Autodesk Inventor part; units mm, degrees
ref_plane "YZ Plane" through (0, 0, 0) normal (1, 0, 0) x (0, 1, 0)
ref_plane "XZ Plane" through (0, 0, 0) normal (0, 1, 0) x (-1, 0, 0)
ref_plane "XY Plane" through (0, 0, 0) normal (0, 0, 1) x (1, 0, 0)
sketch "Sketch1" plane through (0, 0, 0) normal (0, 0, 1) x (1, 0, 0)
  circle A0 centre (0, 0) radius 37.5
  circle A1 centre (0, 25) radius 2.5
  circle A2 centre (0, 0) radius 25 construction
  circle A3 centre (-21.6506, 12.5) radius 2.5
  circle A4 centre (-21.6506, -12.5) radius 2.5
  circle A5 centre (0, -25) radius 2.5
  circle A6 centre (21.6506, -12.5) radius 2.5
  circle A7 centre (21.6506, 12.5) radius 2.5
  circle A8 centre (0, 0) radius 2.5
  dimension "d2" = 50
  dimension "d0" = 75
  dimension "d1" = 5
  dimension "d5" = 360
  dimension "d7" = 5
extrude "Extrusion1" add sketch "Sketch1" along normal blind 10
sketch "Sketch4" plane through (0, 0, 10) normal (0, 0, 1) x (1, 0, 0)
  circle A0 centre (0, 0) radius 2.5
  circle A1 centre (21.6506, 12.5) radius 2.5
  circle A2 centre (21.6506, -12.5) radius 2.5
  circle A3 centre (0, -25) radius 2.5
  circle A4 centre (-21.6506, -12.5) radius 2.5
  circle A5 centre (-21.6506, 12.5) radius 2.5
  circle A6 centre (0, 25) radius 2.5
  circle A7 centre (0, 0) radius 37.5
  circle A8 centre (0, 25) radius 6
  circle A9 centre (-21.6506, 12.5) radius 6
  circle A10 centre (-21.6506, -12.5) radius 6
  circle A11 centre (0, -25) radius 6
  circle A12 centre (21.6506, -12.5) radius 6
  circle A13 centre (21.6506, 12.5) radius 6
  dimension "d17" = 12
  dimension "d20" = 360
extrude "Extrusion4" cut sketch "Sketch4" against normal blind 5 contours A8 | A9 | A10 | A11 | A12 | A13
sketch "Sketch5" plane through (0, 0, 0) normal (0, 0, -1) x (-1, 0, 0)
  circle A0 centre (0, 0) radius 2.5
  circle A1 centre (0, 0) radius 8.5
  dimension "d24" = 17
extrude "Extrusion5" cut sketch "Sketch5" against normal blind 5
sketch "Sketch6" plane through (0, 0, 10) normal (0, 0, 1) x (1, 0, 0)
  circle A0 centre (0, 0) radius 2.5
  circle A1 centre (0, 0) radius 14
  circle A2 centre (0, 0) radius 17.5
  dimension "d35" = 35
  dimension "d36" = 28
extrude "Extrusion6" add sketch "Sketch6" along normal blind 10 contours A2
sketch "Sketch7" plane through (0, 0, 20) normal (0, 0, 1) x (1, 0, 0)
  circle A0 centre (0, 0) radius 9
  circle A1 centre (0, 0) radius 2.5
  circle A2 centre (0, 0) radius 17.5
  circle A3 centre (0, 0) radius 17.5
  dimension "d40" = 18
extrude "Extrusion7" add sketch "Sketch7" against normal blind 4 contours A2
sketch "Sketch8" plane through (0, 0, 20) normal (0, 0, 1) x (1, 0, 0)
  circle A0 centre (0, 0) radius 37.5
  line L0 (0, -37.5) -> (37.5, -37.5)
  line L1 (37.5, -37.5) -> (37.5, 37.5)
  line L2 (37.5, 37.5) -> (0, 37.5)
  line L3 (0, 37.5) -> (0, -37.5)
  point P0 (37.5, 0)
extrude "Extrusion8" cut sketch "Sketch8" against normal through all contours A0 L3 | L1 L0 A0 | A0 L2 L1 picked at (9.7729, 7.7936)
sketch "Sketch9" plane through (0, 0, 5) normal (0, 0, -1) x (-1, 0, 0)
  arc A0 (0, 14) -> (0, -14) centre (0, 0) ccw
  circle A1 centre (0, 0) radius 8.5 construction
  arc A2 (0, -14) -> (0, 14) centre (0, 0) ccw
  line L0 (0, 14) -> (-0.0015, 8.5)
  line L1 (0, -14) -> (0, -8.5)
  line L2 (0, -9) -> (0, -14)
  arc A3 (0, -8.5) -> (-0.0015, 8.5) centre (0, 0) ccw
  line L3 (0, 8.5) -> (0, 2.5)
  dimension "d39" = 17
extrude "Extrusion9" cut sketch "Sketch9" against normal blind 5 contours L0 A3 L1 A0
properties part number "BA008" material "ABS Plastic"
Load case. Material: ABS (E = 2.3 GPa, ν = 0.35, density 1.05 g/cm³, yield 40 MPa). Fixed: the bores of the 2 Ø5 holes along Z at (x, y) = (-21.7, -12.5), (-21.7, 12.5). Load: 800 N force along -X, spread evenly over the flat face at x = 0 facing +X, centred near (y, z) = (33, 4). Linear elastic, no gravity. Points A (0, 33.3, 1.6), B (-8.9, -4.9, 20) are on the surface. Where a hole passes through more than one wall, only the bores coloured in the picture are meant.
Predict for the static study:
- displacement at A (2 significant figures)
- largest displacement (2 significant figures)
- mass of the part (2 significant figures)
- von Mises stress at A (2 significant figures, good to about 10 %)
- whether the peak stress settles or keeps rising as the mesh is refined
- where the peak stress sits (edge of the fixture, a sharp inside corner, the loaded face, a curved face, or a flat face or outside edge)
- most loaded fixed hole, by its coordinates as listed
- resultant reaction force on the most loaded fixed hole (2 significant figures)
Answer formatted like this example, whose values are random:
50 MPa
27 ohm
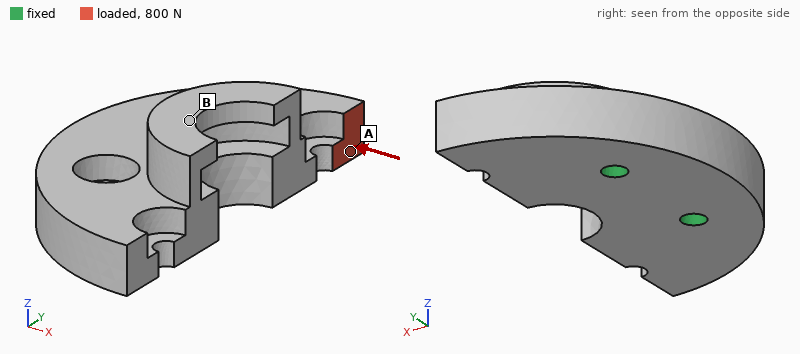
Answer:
0.50 mm
0.61 mm
22 g
10 MPa
keeps rising
edge of the fixture
(-21.7, 12.5)
1.3 kN
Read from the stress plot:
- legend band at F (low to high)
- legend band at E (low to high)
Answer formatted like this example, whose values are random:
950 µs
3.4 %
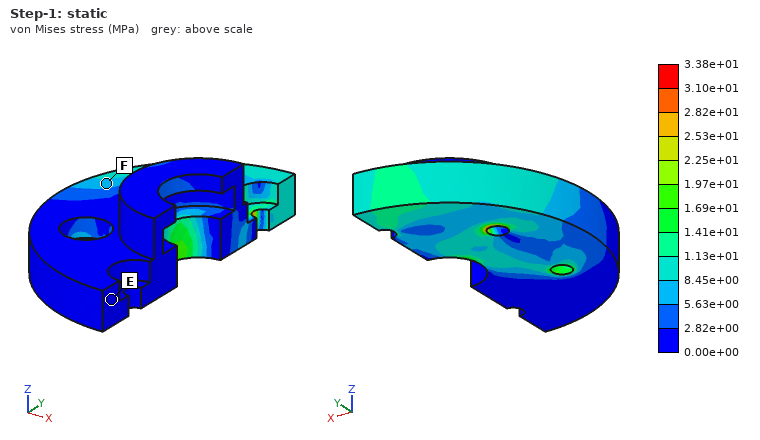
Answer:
5.63e+00 to 8.45e+00 MPa
0.00e+00 to 2.82e+00 MPa
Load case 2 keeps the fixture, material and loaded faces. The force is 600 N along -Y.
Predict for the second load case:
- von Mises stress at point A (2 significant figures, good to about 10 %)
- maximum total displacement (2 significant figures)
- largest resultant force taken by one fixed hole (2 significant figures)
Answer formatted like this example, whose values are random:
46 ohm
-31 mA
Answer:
19 MPa
0.53 mm
560 N
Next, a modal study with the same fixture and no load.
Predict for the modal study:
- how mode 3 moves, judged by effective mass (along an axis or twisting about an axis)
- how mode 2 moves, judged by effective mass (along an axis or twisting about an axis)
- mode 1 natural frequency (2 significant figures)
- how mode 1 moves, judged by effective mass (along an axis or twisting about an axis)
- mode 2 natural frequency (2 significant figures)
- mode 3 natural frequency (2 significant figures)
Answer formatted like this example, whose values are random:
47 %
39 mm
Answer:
along Y
twisting about X
1700 Hz
along Z
2300 Hz
3500 Hz
